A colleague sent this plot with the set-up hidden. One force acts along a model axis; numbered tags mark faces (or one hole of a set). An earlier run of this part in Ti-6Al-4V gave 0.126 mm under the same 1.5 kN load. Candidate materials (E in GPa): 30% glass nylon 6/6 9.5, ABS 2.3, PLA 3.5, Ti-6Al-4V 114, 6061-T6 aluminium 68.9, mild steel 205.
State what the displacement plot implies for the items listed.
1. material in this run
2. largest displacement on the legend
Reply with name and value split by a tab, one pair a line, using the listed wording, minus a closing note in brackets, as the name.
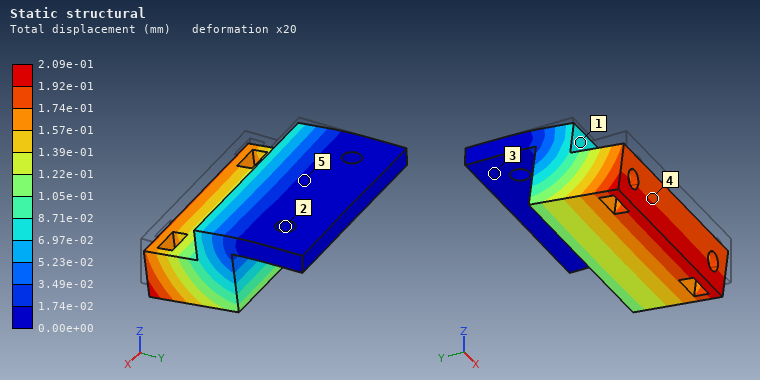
material in this run	6061-T6 aluminium
largest displacement on the legend	2.09e-01 mm
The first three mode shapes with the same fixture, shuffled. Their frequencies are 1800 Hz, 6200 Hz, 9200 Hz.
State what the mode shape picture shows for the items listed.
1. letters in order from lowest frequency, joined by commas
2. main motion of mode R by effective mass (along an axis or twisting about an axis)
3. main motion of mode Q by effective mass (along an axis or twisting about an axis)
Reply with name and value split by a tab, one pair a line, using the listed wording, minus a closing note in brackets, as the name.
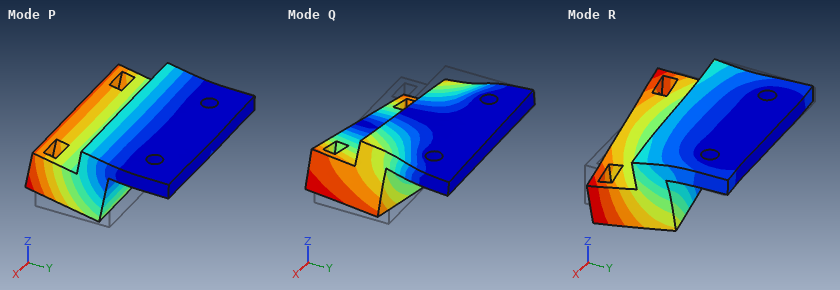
letters in order from lowest frequency, joined by commas	P, Q, R
main motion of mode R by effective mass	along X
main motion of mode Q by effective mass	along X
